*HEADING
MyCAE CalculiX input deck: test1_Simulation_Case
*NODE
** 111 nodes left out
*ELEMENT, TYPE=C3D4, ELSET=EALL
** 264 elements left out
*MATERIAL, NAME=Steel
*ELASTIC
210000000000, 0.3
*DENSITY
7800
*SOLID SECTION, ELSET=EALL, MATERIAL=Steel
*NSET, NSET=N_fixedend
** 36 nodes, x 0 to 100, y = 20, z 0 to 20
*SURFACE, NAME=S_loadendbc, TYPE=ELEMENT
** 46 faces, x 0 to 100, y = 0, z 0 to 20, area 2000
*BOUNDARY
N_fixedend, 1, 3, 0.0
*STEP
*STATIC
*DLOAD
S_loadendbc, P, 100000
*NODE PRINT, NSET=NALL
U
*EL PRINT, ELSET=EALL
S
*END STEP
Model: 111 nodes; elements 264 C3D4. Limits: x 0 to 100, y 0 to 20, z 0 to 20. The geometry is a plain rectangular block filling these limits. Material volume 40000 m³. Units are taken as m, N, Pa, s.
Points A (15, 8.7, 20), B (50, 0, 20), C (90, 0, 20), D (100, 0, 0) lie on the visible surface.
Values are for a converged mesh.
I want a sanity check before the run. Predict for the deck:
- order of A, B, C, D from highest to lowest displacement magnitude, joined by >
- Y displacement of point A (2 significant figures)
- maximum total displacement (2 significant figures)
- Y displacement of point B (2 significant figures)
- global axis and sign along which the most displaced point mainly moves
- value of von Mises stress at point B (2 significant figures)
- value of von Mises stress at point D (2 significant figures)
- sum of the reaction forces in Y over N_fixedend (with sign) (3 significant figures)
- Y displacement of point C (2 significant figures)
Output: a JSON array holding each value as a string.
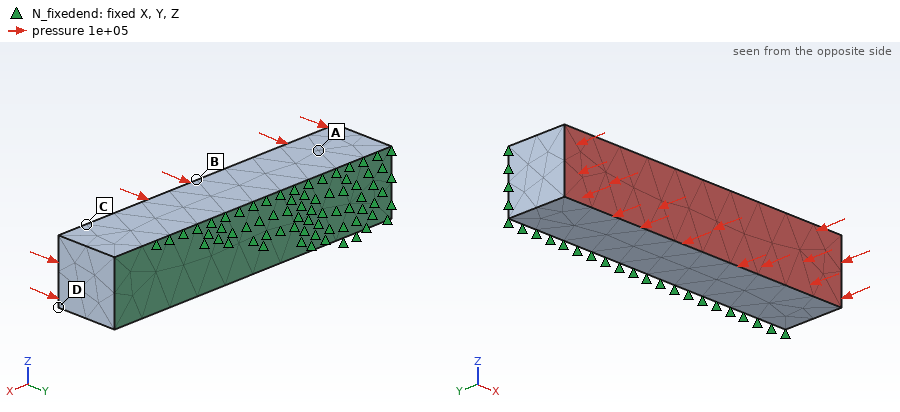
["D > C > B > A", "4.9e-06 m", "1.1e-05 m", "8.5e-06 m", "+Y", "91000 Pa", "100000 Pa", "-2.00e+08 N", "9.1e-06 m"]
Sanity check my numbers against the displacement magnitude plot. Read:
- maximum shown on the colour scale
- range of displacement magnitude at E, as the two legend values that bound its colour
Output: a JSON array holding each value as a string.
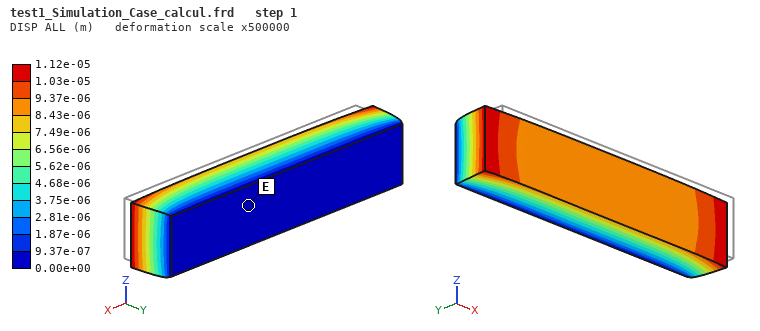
["1.12e-05 m", "0.00e+00 to 9.37e-07 m"]
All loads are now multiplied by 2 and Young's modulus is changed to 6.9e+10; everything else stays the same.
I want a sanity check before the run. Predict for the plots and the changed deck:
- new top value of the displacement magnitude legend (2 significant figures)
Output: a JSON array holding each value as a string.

["6.8e-05 m"]
